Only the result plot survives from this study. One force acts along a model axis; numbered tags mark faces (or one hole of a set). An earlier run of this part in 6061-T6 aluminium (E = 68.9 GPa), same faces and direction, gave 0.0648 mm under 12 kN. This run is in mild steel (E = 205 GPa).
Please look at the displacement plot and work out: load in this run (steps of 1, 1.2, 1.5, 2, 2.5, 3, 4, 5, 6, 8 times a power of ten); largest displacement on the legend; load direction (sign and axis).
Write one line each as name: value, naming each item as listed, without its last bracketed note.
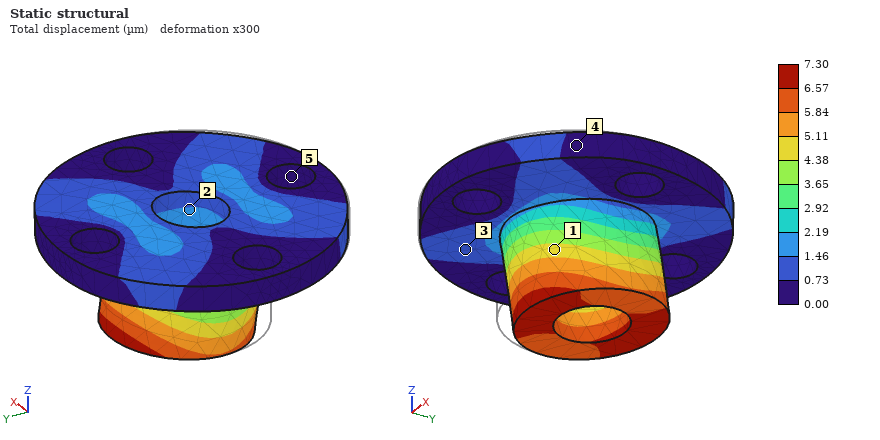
load in this run: 4 kN
largest displacement on the legend: 7.30 µm
load direction: +Y
